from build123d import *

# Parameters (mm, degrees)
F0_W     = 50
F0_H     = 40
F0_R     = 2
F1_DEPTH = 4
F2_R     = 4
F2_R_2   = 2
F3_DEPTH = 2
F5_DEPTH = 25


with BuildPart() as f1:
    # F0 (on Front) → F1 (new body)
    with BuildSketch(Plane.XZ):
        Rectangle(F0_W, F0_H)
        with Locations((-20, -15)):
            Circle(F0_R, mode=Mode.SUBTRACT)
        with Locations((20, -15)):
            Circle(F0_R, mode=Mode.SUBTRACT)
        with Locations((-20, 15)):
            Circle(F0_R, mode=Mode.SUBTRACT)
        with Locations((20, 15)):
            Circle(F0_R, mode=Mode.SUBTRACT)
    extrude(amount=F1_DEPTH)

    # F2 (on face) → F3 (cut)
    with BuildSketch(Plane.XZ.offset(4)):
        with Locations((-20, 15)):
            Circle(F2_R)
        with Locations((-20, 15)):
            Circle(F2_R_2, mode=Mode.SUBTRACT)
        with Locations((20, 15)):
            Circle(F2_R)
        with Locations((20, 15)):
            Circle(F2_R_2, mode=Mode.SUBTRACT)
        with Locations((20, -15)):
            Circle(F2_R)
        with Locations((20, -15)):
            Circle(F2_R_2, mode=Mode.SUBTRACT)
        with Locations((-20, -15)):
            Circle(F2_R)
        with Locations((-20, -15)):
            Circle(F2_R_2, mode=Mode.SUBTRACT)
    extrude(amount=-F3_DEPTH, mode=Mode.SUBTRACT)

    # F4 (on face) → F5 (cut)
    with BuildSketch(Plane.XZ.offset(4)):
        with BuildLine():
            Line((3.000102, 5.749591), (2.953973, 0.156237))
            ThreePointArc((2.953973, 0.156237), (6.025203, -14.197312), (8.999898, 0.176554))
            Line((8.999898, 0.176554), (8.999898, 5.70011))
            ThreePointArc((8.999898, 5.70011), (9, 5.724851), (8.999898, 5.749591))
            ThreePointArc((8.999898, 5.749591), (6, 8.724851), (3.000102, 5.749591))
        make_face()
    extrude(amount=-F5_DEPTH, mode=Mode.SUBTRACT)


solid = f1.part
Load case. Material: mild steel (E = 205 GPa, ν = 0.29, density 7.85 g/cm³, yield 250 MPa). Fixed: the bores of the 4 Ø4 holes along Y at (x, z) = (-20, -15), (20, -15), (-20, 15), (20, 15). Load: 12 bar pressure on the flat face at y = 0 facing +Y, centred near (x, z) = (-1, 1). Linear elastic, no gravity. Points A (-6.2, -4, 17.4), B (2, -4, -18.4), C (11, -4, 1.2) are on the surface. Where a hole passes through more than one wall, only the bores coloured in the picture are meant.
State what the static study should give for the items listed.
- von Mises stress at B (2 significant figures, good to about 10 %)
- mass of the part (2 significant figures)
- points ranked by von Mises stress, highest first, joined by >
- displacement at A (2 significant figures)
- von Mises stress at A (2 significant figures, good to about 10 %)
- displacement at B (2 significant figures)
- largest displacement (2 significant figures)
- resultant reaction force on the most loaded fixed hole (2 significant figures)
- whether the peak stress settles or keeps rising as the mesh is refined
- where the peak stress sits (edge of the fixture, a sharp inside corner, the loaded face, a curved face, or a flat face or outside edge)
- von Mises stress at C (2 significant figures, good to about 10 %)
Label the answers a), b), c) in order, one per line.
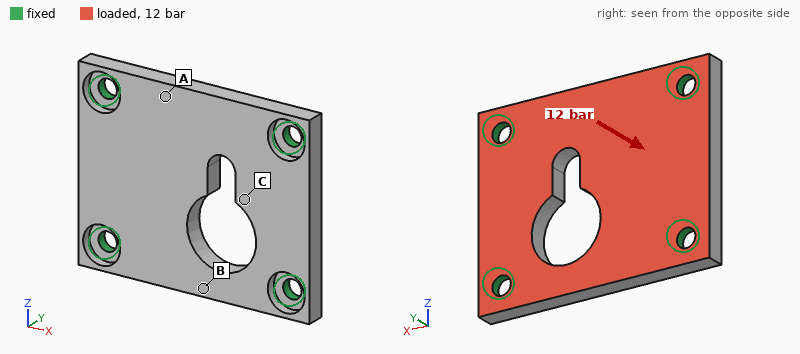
a) 60 MPa
b) 52 g
c) B > A > C
d) 11 µm
e) 41 MPa
f) 13 µm
g) 23 µm
h) 680 N
i) keeps rising
j) edge of the fixture
k) 18 MPa
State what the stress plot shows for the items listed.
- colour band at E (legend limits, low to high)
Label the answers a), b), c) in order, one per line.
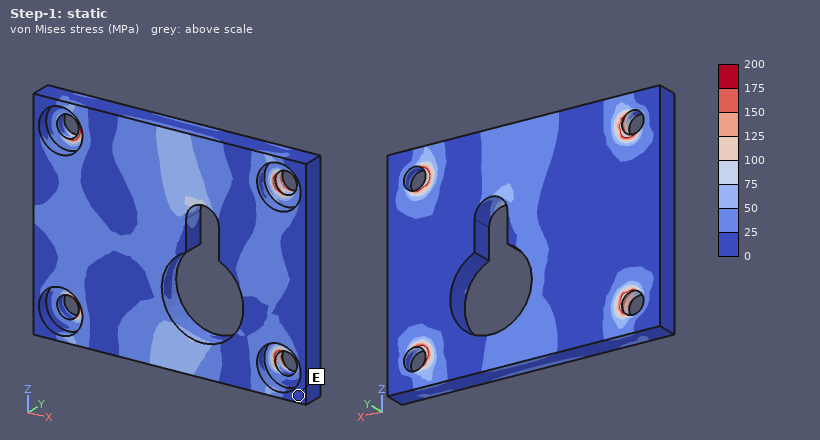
a) 0 to 25 MPa
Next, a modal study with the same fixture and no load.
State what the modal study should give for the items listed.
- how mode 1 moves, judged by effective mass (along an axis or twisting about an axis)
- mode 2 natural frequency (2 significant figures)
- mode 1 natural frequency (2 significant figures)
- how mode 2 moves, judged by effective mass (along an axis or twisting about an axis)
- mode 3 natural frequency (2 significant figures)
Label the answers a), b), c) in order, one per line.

a) along Y
b) 13 kHz
c) 8600 Hz
d) twisting about X
e) 16 kHz
